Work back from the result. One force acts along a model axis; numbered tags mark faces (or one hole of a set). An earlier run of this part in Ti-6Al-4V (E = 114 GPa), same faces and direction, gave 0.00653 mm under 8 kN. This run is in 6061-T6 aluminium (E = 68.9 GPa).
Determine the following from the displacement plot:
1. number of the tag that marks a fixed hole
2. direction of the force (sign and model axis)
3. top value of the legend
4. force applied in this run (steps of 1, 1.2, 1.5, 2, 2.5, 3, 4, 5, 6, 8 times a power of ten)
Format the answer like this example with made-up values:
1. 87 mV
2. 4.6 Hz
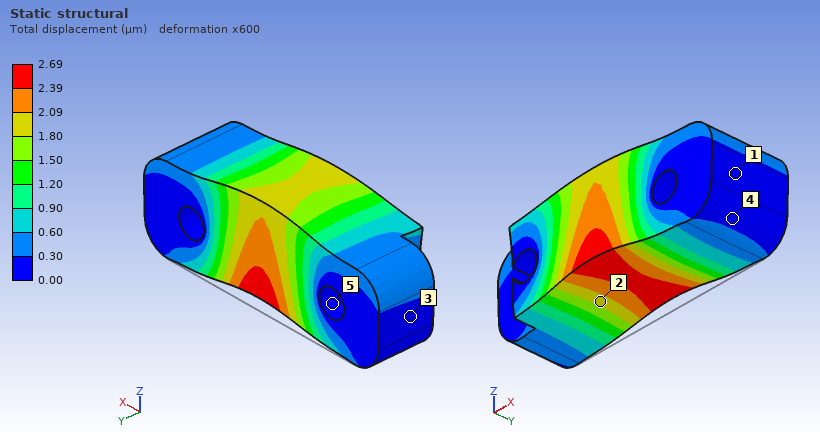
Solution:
1. 5
2. +Z
3. 2.69 µm
4. 2 kN
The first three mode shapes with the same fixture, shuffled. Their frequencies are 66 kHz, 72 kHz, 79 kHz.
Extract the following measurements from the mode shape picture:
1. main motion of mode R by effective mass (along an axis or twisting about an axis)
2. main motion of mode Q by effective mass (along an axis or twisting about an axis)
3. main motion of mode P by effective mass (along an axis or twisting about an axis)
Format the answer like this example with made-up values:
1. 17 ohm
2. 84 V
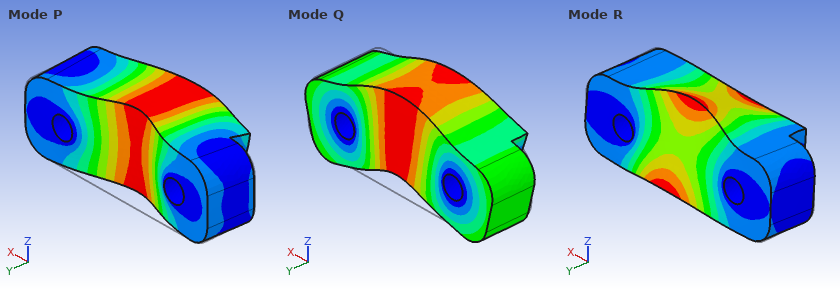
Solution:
1. twisting about X
2. along Z
3. along Y
